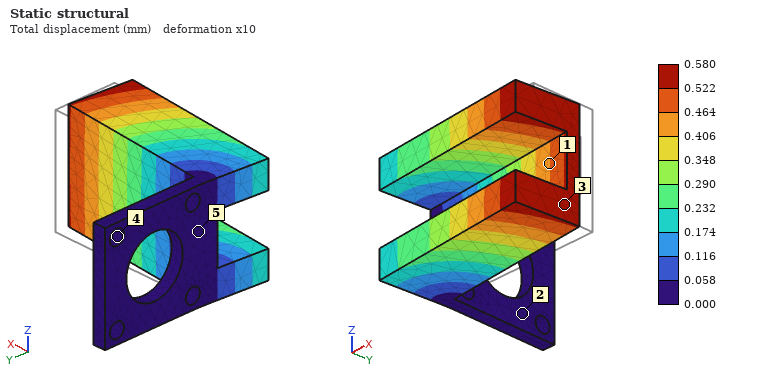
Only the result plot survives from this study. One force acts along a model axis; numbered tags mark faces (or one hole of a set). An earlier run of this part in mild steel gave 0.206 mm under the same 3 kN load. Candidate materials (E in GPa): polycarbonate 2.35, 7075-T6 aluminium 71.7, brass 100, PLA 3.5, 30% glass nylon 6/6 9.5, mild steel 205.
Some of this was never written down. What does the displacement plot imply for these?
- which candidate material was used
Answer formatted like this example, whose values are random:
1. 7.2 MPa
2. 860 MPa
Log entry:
1. 7075-T6 aluminium
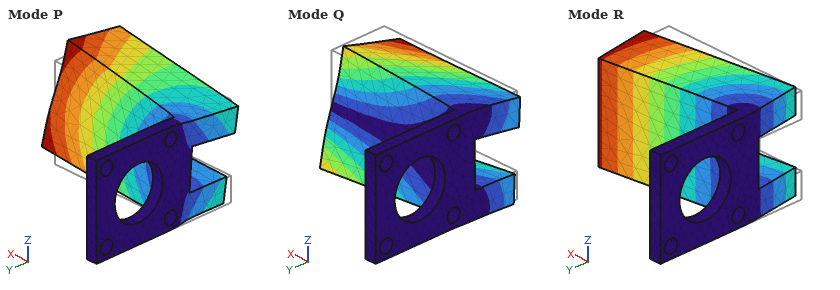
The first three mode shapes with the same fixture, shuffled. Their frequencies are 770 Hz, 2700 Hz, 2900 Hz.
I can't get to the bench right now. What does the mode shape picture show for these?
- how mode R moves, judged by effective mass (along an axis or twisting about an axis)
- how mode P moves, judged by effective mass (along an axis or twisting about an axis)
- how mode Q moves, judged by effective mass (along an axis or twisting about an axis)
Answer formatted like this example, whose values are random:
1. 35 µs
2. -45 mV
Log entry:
1. along Y
2. along Z
3. along Z
